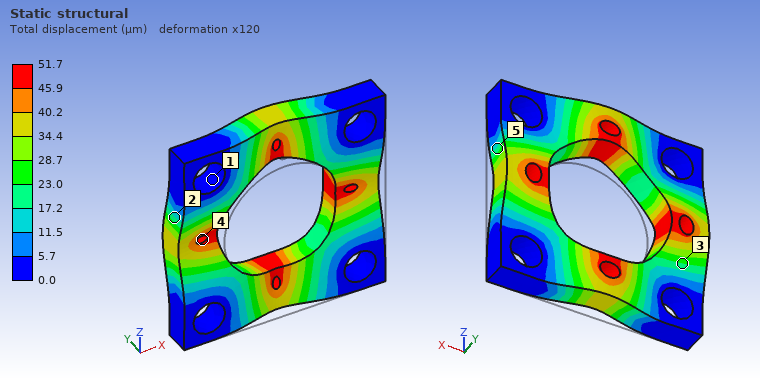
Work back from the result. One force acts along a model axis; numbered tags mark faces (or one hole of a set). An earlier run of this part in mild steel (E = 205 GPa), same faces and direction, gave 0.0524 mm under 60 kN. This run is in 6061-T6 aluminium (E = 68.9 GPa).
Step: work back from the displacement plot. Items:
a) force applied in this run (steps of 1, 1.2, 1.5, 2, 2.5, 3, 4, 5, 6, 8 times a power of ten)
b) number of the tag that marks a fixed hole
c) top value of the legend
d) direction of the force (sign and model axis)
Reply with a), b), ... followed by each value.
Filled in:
a) 20 kN
b) 1
c) 51.7 µm
d) +Y
